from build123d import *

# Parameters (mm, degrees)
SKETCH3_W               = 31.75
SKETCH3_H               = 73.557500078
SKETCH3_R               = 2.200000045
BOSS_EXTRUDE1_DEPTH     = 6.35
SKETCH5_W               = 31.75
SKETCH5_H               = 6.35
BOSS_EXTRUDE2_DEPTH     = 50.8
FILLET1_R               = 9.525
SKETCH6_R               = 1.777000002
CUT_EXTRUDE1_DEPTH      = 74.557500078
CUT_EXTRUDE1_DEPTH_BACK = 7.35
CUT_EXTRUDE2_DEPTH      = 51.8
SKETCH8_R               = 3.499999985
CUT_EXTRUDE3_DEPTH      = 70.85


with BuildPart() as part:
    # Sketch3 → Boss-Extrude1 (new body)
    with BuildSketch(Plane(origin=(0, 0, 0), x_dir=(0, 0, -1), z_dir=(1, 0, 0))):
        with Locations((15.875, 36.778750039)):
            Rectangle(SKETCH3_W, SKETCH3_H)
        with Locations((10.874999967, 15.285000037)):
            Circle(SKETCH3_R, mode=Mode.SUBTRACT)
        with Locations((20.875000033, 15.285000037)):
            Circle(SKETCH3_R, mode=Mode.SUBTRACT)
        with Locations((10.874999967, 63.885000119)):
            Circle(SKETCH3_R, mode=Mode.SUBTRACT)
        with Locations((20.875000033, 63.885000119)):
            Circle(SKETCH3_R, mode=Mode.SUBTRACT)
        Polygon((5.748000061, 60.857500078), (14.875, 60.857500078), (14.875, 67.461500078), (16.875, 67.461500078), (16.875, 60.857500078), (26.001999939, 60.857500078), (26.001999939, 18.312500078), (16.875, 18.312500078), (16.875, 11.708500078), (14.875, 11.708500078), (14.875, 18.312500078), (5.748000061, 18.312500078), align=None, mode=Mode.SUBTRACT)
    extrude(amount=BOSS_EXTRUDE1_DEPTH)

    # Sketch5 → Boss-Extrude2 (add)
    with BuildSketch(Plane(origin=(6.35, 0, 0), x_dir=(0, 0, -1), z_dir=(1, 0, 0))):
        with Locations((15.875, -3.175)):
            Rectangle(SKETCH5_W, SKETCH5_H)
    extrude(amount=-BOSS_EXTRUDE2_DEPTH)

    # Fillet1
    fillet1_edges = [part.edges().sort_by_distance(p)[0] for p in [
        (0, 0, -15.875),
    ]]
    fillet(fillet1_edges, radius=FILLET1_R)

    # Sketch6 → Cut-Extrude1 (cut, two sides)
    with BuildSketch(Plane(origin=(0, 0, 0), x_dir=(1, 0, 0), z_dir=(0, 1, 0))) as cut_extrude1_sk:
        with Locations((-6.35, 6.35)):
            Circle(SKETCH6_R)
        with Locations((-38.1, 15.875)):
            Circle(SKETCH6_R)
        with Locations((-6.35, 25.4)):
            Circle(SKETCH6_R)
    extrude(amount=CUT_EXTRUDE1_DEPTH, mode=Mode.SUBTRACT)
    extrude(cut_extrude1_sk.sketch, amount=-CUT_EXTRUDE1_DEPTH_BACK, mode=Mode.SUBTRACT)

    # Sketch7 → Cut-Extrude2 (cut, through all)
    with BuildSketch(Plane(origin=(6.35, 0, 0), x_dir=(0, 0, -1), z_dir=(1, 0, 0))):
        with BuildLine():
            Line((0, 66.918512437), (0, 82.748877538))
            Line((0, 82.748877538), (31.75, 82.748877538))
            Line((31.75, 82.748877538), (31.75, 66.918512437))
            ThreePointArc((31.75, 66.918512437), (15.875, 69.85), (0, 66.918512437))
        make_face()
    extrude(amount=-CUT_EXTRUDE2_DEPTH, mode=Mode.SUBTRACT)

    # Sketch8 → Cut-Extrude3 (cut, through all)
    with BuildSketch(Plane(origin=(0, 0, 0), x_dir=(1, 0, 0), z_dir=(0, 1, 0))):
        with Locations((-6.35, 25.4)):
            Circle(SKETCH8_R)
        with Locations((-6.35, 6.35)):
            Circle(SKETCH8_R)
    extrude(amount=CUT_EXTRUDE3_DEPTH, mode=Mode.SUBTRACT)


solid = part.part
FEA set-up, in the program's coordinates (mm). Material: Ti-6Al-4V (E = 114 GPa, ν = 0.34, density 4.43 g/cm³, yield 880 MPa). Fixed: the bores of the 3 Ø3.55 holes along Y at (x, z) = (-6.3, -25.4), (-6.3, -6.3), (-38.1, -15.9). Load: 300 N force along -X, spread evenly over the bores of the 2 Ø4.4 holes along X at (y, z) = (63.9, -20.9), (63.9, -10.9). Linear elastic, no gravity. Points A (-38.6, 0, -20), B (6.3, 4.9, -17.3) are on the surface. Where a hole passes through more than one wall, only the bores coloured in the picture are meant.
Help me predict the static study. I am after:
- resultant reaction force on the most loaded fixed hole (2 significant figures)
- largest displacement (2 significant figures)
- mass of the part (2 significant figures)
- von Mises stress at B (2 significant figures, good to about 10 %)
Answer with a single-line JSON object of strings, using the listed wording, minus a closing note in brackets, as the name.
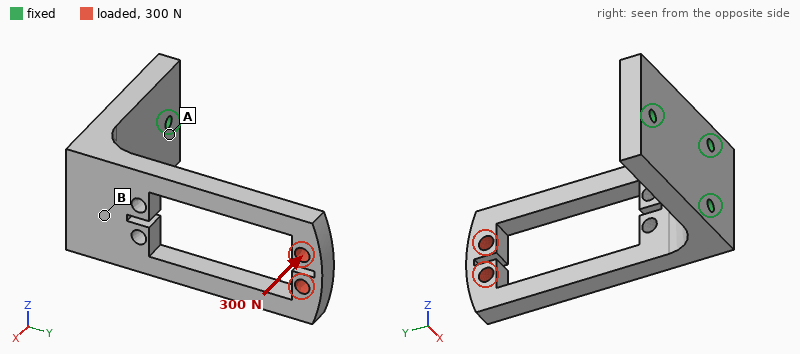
{"resultant reaction force on the most loaded fixed hole": "170 N", "largest displacement": "0.80 mm", "mass of the part": "82 g", "von Mises stress at B": "46 MPa"}
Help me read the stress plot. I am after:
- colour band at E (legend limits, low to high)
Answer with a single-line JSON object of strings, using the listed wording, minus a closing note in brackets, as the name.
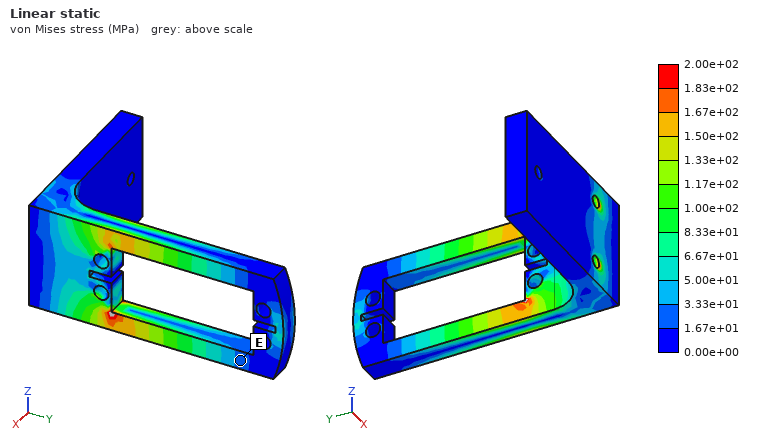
{"colour band at E": "1.67e+01 to 3.33e+01 MPa"}
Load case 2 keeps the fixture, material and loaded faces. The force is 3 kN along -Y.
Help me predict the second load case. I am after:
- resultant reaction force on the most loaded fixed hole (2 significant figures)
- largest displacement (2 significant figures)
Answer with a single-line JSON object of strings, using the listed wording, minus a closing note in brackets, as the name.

{"resultant reaction force on the most loaded fixed hole": "1.6 kN", "largest displacement": "0.18 mm"}
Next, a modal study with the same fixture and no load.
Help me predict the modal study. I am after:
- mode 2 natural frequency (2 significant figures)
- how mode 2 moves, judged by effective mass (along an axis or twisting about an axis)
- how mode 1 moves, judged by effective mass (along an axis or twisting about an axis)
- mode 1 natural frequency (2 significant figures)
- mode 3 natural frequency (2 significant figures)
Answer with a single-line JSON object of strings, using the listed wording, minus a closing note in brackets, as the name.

{"mode 2 natural frequency": "1900 Hz", "how mode 2 moves, judged by effective mass": "along Z", "how mode 1 moves, judged by effective mass": "along X", "mode 1 natural frequency": "1100 Hz", "mode 3 natural frequency": "3000 Hz"}
